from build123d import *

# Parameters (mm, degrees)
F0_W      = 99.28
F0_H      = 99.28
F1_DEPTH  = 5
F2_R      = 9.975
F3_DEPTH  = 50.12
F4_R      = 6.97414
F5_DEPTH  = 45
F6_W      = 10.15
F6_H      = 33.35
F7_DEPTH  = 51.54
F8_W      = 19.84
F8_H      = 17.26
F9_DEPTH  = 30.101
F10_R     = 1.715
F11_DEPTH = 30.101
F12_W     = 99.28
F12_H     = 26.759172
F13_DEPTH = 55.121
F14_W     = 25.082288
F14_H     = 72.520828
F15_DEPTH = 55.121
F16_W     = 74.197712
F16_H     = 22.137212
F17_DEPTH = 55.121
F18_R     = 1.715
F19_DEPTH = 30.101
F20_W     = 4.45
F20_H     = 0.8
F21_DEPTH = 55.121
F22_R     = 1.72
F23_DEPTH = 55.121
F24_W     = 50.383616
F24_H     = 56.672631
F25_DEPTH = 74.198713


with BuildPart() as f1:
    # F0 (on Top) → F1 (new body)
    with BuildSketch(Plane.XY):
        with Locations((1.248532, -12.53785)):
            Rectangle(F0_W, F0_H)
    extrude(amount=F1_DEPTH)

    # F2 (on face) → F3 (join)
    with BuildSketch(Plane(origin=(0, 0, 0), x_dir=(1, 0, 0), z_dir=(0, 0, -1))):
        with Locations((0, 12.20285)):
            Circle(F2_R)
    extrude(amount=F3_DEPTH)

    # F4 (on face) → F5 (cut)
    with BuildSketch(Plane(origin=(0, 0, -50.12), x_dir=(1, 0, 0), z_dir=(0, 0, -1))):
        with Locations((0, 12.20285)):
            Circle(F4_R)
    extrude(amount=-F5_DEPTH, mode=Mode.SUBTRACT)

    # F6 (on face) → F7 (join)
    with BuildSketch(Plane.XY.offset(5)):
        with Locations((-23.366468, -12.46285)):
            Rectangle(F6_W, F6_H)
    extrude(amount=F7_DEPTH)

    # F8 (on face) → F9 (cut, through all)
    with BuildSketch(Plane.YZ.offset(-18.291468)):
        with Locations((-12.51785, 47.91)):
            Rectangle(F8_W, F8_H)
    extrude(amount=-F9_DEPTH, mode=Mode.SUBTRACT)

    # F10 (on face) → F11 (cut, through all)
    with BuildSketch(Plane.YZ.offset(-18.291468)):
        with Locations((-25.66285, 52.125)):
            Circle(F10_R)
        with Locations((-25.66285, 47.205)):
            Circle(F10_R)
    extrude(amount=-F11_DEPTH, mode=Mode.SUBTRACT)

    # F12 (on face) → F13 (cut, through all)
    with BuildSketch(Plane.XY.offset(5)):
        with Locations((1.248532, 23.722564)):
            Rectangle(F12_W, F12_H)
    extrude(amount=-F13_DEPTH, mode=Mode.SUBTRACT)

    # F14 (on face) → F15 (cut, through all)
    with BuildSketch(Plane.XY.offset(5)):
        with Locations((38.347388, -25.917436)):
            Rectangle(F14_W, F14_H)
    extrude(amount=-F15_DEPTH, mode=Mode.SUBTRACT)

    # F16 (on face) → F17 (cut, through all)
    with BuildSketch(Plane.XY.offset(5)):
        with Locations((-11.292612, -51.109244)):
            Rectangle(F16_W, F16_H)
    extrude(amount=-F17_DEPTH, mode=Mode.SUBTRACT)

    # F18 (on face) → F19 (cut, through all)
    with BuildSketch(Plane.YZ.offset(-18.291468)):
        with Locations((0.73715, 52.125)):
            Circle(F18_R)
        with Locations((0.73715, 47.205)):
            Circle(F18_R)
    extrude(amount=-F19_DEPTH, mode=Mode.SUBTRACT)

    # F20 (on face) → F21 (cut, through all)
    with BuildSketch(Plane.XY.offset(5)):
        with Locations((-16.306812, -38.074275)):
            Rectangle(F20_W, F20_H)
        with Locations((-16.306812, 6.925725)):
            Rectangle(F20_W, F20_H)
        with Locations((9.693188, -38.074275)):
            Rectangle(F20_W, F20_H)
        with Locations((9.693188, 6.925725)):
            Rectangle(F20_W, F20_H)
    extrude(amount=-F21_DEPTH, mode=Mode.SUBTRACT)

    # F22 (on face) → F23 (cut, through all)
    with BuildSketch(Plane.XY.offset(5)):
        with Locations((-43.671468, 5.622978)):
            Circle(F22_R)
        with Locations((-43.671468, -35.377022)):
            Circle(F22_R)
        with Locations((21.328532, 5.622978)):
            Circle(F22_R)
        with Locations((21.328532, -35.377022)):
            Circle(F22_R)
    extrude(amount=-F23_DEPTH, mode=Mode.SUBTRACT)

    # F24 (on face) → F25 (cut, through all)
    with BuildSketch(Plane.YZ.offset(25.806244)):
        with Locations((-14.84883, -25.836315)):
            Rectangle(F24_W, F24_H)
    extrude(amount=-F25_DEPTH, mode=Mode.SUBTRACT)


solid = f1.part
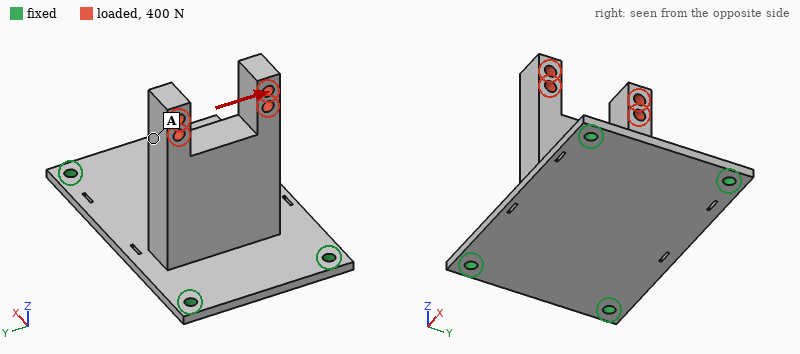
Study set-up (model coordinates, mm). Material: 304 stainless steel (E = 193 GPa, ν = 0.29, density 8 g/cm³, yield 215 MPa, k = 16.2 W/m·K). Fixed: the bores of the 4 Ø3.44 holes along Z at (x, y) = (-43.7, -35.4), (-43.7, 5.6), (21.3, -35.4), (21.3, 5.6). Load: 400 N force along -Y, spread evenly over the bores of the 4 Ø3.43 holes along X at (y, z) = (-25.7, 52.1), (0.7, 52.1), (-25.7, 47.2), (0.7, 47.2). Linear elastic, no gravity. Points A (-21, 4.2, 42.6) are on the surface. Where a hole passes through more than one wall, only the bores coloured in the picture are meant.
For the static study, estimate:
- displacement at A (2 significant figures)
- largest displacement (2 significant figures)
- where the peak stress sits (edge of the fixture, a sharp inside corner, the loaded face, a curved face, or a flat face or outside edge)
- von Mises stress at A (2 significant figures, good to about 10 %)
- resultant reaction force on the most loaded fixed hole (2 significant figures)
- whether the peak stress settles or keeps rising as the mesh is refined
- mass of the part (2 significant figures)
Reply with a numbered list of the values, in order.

1. 0.12 mm
2. 0.16 mm
3. edge of the fixture
4. 20 MPa
5. 470 N
6. keeps rising
7. 180 g
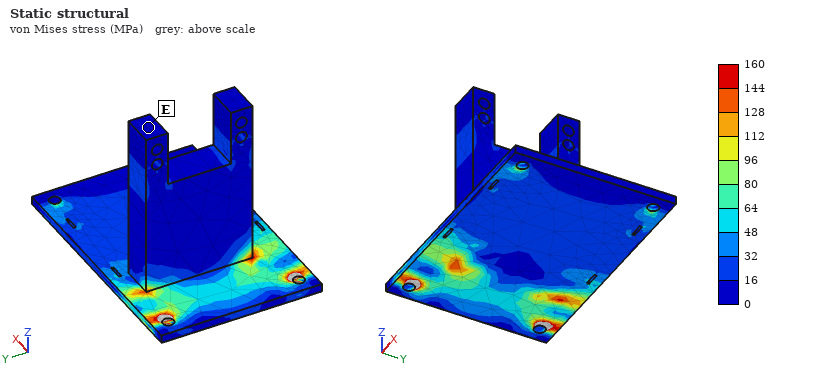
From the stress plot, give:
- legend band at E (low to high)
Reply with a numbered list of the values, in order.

1. 0 to 16 MPa
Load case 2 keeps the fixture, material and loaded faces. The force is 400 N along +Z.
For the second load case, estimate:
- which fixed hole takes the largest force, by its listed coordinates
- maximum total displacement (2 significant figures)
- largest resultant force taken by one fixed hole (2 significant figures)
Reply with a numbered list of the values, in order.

1. (-43.7, 5.6)
2. 68 µm
3. 170 N
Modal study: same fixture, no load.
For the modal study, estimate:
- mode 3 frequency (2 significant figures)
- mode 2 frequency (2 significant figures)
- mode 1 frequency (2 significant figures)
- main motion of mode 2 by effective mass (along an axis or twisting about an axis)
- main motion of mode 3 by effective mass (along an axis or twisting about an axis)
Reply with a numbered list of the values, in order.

1. 2100 Hz
2. 1400 Hz
3. 950 Hz
4. along Y
5. along Z
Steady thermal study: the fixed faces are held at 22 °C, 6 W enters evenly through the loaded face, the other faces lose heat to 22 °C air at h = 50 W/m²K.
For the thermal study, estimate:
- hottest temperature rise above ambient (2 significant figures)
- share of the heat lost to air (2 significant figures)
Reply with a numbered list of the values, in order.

1. 48 K
2. 92 %
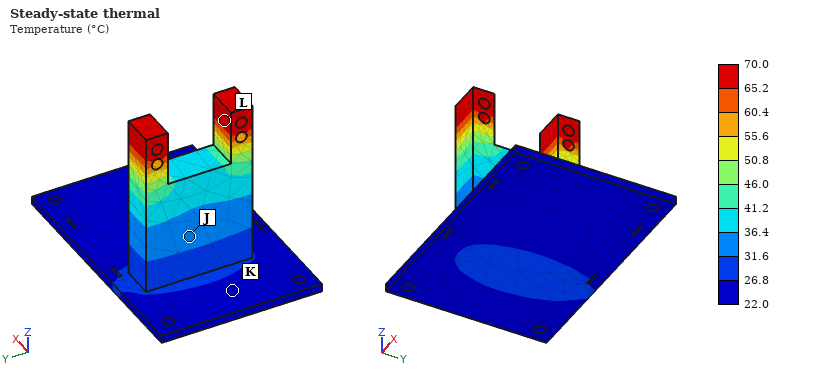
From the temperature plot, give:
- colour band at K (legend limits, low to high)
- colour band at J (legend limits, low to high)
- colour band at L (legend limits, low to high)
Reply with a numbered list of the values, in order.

1. 22.0 to 26.8 °C
2. 31.6 to 36.4 °C
3. 65.2 to 70.0 °C
